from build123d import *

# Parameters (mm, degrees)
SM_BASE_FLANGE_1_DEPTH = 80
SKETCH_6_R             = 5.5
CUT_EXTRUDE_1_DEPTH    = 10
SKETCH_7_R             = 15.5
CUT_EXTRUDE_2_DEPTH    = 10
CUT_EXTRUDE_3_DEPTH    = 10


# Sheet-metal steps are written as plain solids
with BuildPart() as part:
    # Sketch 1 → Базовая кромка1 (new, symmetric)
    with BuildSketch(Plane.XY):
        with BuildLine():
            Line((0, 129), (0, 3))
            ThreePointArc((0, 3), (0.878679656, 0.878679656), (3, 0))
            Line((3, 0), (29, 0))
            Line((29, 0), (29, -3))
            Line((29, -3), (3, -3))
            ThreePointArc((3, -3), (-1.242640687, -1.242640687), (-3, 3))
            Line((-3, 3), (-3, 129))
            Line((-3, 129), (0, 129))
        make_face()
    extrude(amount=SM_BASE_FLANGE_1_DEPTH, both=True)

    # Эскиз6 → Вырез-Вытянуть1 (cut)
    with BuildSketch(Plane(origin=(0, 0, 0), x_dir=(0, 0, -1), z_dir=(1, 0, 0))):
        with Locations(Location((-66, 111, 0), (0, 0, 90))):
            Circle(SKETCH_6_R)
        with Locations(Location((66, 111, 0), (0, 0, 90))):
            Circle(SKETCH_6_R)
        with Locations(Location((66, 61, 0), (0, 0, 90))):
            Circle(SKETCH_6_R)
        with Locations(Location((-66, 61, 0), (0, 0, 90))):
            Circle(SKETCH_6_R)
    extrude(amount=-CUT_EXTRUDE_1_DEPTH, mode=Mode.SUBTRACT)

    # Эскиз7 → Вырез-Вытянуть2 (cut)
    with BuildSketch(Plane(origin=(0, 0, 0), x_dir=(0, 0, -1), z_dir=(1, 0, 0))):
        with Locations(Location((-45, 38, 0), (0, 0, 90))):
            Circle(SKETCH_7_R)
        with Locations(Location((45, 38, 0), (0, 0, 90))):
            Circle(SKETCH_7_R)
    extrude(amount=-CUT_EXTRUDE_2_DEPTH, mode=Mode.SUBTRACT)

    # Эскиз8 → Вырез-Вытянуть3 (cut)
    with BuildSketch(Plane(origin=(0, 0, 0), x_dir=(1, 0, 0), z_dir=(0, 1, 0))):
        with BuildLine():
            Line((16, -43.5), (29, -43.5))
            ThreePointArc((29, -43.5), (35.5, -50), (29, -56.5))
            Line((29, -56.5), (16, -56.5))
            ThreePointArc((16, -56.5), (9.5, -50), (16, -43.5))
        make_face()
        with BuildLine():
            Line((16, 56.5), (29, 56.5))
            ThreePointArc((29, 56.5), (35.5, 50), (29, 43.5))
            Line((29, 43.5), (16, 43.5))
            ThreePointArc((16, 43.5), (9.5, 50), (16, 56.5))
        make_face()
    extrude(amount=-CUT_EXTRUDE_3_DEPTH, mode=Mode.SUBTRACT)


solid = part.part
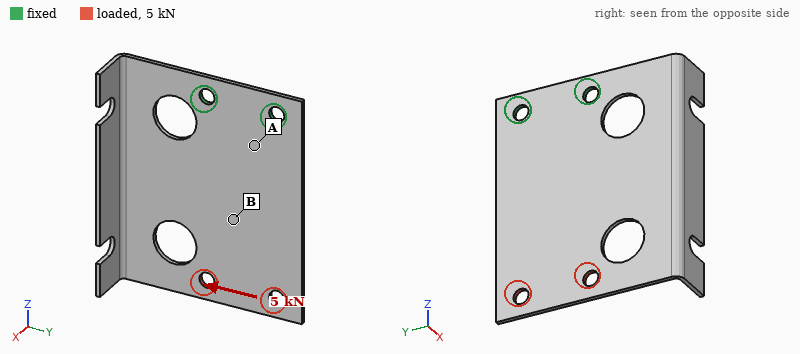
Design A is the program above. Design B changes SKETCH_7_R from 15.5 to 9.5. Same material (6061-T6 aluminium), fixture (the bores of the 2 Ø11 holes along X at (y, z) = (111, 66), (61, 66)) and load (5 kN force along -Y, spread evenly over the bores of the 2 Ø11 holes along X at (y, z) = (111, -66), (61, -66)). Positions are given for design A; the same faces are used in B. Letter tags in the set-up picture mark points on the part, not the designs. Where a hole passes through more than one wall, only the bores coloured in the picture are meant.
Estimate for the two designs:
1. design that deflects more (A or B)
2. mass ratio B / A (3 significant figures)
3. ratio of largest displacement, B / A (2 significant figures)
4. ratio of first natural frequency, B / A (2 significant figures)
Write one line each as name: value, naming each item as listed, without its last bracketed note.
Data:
design that deflects more: A
mass ratio B / A: 1.04
ratio of largest displacement, B / A: 0.89
ratio of first natural frequency, B / A: 1.0
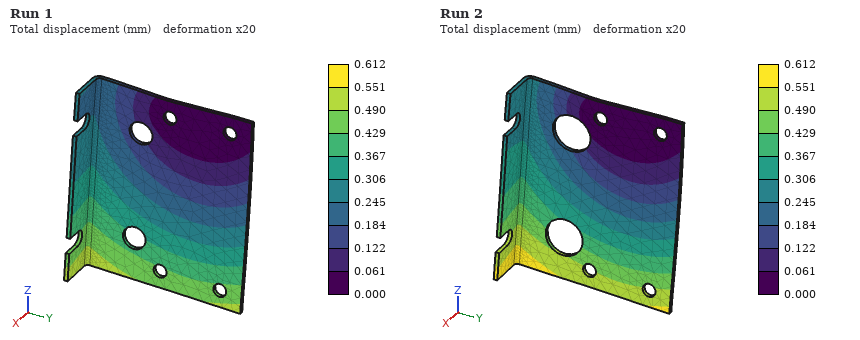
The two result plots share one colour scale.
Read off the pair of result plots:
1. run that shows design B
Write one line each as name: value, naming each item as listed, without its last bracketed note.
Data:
run that shows design B: Run 1
